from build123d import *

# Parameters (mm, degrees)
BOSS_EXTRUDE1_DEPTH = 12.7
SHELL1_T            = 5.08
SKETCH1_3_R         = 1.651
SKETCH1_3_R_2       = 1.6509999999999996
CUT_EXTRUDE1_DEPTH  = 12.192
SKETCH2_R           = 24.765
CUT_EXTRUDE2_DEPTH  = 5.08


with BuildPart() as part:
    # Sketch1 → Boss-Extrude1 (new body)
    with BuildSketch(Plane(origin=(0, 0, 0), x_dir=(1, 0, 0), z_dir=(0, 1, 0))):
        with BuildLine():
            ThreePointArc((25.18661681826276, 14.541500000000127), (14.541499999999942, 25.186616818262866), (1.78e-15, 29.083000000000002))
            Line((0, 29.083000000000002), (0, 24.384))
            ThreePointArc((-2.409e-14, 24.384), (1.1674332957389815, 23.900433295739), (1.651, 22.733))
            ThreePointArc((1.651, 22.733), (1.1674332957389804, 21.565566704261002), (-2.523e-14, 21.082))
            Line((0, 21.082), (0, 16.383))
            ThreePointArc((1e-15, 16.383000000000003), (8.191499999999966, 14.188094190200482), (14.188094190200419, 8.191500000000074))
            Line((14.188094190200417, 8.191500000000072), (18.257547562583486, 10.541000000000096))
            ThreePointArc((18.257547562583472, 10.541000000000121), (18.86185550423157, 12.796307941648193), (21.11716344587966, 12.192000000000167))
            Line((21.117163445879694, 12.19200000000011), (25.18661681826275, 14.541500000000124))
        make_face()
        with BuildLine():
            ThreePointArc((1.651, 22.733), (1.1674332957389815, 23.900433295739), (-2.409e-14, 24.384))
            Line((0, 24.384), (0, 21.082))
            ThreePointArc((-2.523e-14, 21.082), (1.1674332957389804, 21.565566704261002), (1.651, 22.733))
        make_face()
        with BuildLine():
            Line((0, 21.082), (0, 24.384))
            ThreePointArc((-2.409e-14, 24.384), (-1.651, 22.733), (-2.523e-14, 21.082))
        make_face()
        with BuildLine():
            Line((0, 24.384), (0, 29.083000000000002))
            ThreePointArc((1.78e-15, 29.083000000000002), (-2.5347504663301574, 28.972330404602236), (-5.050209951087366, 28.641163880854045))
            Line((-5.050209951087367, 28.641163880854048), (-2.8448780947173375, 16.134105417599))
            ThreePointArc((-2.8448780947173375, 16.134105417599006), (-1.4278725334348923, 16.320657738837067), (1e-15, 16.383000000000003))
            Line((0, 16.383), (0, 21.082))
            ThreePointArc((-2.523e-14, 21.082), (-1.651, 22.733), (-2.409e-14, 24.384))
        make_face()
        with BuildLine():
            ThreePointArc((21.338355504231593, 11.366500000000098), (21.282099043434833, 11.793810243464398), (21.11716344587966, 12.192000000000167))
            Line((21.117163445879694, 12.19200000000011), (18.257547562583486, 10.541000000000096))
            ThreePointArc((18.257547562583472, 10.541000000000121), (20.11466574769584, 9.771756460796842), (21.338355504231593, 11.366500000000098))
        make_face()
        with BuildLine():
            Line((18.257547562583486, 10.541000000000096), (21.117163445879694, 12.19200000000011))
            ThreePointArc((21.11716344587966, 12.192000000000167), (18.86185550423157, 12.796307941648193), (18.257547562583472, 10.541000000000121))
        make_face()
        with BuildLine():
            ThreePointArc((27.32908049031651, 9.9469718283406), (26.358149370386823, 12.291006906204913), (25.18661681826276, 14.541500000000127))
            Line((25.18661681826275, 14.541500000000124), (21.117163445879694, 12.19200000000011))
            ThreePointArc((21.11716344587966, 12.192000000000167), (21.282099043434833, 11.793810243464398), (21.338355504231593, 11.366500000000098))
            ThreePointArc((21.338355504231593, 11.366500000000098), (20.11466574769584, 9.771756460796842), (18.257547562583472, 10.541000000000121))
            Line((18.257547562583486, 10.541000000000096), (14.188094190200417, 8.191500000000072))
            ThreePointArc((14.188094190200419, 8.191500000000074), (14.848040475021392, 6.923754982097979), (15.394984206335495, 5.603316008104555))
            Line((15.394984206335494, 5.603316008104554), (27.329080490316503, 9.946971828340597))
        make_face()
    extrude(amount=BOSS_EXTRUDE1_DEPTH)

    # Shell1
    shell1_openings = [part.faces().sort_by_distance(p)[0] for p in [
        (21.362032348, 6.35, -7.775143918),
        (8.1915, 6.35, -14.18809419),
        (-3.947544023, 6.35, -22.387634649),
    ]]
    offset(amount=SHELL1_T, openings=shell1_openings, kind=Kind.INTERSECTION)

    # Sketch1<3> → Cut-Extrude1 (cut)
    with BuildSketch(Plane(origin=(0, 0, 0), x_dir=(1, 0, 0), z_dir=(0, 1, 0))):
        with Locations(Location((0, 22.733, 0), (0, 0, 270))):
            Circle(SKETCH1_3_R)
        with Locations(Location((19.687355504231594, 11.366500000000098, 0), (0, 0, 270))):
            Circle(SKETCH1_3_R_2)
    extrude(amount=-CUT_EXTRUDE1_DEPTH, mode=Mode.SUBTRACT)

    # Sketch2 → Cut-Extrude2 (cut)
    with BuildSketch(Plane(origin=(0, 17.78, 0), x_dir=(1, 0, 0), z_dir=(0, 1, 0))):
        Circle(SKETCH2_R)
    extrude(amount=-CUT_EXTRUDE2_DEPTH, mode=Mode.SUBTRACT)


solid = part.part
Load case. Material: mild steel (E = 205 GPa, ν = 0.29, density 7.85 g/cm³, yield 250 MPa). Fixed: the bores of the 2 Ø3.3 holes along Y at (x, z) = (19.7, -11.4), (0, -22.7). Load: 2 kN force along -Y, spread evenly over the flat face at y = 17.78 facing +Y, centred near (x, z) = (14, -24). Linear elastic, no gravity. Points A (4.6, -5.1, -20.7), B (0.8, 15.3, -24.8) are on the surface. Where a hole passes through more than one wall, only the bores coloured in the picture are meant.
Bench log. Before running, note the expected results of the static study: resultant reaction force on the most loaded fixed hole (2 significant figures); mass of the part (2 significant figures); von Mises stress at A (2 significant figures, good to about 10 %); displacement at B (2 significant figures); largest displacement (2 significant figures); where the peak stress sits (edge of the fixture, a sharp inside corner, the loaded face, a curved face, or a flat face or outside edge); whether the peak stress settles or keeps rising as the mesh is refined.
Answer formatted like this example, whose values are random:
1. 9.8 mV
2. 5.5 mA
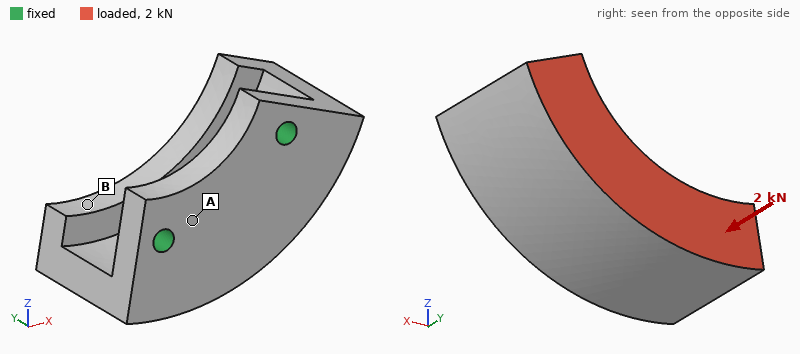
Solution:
1. 1.0 kN
2. 62 g
3. 40 MPa
4. 15 µm
5. 20 µm
6. edge of the fixture
7. keeps rising
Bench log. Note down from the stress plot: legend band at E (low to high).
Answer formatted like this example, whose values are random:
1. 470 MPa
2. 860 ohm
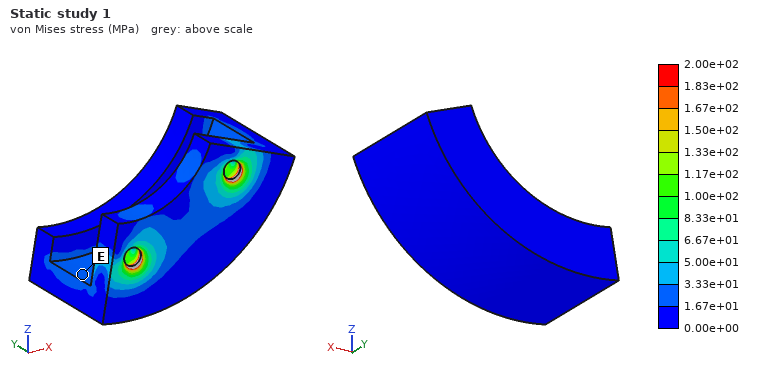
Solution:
1. 1.67e+01 to 3.33e+01 MPa
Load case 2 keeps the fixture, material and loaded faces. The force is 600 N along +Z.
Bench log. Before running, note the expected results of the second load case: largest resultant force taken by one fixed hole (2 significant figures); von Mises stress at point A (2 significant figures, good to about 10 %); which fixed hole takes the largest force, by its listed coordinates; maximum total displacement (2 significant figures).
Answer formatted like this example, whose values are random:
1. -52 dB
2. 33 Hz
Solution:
1. 440 N
2. 41 MPa
3. (19.7, -11.4)
4. 40 µm
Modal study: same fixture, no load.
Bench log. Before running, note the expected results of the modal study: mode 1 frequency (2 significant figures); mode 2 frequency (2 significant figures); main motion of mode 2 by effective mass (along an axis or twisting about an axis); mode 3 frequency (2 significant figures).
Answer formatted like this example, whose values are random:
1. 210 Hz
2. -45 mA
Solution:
1. 4500 Hz
2. 8100 Hz
3. along X
4. 14 kHz
